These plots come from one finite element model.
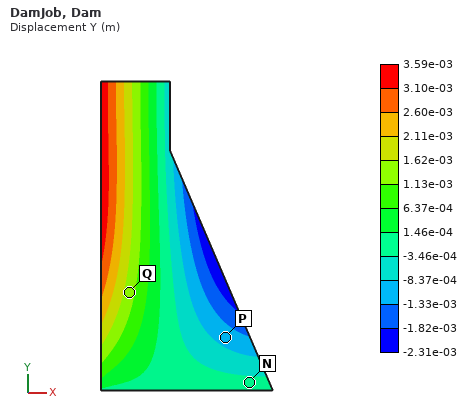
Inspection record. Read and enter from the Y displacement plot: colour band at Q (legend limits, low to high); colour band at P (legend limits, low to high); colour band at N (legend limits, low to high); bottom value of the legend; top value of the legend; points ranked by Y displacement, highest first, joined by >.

1.13e-03 to 1.62e-03 m
-1.33e-03 to -8.37e-04 m
-3.46e-04 to 1.46e-04 m
-2.31e-03 m
3.59e-03 m
Q > N > P
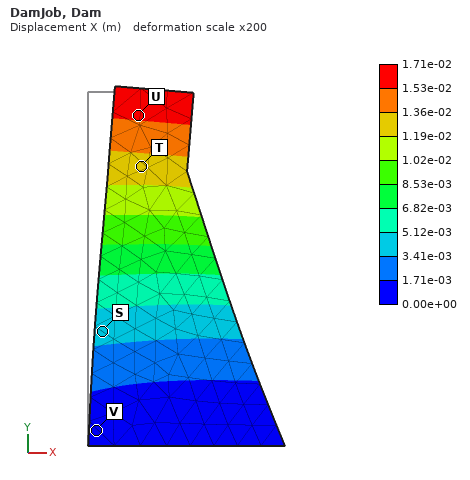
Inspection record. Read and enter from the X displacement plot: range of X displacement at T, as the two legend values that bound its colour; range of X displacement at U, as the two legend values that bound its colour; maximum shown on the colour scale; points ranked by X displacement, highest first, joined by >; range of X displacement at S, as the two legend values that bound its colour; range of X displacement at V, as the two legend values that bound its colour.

1.19e-02 to 1.36e-02 m
1.53e-02 to 1.71e-02 m
1.71e-02 m
U > T > S > V
3.41e-03 to 5.12e-03 m
0.00e+00 to 1.71e-03 m
